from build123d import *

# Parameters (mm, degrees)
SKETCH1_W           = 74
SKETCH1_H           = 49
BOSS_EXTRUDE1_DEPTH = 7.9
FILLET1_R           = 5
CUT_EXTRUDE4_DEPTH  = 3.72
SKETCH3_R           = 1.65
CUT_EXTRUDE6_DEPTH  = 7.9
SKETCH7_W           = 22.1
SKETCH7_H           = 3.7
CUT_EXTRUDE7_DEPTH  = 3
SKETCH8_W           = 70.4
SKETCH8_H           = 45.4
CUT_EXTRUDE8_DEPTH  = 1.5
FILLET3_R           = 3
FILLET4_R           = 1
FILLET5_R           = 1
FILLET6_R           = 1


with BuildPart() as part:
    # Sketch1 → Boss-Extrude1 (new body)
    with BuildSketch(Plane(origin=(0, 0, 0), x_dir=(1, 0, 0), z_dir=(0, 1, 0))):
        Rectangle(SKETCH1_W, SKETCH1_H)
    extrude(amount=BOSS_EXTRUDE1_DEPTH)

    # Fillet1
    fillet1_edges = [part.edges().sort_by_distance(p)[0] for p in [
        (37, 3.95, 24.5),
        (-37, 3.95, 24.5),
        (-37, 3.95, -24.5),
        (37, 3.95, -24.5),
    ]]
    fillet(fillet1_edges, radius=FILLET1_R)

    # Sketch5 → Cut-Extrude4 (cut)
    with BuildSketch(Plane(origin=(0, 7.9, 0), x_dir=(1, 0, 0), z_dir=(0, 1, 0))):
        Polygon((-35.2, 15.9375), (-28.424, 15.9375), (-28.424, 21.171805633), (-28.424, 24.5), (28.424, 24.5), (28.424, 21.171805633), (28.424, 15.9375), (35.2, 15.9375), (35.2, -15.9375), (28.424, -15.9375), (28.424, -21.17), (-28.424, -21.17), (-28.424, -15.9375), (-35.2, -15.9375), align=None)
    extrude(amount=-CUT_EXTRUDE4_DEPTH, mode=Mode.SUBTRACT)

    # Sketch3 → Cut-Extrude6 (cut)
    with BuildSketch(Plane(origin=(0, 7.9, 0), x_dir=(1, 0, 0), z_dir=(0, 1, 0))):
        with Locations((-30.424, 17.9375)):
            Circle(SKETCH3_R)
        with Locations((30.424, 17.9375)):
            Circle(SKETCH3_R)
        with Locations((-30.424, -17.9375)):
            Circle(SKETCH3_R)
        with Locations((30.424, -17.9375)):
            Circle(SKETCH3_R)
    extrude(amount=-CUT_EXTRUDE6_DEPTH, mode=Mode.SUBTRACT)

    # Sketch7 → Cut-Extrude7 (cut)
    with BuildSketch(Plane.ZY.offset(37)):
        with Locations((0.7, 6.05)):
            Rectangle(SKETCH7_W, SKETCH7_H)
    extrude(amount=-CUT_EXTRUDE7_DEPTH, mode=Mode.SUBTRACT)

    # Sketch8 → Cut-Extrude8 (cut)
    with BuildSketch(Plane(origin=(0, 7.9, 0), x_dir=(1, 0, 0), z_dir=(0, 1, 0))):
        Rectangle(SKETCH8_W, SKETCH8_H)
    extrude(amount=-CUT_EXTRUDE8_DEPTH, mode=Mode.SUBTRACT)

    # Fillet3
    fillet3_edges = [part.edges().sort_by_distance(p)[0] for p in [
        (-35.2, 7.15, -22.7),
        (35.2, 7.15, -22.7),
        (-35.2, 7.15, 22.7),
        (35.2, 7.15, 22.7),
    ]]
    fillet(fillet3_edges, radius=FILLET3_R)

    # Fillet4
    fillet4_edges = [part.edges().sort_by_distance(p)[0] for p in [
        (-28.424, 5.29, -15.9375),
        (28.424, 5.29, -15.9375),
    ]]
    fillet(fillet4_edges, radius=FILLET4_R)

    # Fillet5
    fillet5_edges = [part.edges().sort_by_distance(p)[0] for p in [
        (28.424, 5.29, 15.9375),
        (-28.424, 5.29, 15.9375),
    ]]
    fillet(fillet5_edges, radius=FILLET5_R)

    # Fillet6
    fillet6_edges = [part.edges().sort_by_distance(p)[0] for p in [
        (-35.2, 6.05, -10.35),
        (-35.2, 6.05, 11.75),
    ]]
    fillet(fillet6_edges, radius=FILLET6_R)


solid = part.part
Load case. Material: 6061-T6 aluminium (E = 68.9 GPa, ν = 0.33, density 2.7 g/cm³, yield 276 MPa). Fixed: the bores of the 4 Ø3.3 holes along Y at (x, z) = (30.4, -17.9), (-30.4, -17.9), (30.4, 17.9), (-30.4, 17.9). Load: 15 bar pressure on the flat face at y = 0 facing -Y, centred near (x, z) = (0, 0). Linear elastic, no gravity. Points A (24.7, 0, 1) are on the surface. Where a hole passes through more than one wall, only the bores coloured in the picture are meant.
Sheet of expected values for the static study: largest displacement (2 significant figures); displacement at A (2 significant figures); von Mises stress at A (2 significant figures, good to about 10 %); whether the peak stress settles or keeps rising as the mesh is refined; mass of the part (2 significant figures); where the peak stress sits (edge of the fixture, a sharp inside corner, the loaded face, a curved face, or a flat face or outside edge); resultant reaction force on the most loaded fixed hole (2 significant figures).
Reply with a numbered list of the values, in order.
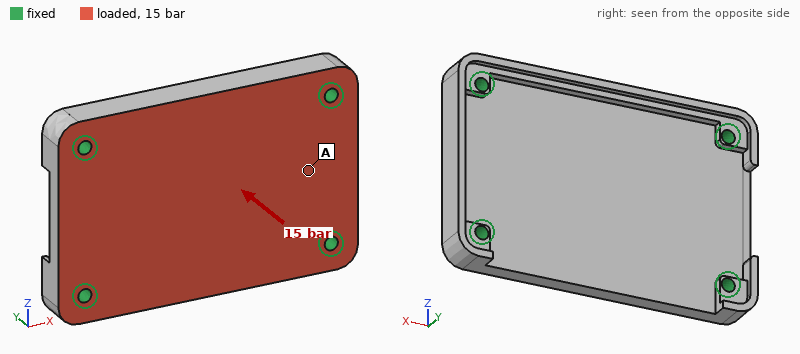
1. 0.16 mm
2. 0.051 mm
3. 39 MPa
4. keeps rising
5. 44 g
6. edge of the fixture
7. 1.4 kN
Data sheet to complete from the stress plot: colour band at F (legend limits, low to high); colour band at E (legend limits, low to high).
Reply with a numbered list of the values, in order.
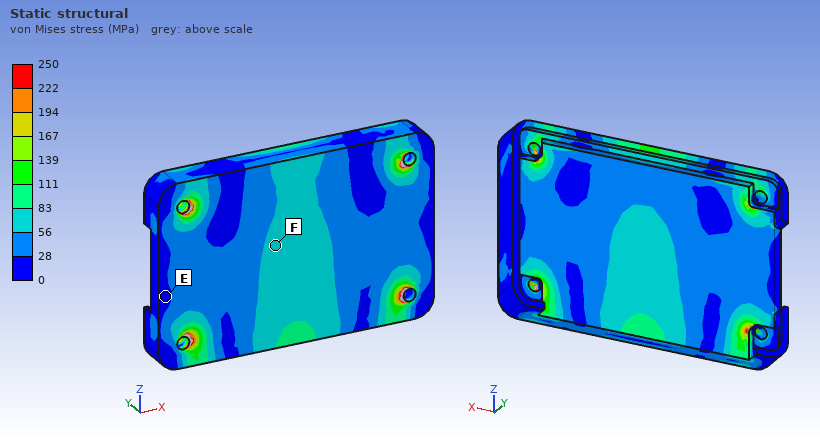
1. 56 to 83 MPa
2. 0 to 28 MPa
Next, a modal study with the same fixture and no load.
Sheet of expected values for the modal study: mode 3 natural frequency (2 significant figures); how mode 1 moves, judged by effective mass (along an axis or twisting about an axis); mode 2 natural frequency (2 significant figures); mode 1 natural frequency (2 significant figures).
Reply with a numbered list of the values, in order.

1. 13 kHz
2. along Y
3. 8000 Hz
4. 5500 Hz
